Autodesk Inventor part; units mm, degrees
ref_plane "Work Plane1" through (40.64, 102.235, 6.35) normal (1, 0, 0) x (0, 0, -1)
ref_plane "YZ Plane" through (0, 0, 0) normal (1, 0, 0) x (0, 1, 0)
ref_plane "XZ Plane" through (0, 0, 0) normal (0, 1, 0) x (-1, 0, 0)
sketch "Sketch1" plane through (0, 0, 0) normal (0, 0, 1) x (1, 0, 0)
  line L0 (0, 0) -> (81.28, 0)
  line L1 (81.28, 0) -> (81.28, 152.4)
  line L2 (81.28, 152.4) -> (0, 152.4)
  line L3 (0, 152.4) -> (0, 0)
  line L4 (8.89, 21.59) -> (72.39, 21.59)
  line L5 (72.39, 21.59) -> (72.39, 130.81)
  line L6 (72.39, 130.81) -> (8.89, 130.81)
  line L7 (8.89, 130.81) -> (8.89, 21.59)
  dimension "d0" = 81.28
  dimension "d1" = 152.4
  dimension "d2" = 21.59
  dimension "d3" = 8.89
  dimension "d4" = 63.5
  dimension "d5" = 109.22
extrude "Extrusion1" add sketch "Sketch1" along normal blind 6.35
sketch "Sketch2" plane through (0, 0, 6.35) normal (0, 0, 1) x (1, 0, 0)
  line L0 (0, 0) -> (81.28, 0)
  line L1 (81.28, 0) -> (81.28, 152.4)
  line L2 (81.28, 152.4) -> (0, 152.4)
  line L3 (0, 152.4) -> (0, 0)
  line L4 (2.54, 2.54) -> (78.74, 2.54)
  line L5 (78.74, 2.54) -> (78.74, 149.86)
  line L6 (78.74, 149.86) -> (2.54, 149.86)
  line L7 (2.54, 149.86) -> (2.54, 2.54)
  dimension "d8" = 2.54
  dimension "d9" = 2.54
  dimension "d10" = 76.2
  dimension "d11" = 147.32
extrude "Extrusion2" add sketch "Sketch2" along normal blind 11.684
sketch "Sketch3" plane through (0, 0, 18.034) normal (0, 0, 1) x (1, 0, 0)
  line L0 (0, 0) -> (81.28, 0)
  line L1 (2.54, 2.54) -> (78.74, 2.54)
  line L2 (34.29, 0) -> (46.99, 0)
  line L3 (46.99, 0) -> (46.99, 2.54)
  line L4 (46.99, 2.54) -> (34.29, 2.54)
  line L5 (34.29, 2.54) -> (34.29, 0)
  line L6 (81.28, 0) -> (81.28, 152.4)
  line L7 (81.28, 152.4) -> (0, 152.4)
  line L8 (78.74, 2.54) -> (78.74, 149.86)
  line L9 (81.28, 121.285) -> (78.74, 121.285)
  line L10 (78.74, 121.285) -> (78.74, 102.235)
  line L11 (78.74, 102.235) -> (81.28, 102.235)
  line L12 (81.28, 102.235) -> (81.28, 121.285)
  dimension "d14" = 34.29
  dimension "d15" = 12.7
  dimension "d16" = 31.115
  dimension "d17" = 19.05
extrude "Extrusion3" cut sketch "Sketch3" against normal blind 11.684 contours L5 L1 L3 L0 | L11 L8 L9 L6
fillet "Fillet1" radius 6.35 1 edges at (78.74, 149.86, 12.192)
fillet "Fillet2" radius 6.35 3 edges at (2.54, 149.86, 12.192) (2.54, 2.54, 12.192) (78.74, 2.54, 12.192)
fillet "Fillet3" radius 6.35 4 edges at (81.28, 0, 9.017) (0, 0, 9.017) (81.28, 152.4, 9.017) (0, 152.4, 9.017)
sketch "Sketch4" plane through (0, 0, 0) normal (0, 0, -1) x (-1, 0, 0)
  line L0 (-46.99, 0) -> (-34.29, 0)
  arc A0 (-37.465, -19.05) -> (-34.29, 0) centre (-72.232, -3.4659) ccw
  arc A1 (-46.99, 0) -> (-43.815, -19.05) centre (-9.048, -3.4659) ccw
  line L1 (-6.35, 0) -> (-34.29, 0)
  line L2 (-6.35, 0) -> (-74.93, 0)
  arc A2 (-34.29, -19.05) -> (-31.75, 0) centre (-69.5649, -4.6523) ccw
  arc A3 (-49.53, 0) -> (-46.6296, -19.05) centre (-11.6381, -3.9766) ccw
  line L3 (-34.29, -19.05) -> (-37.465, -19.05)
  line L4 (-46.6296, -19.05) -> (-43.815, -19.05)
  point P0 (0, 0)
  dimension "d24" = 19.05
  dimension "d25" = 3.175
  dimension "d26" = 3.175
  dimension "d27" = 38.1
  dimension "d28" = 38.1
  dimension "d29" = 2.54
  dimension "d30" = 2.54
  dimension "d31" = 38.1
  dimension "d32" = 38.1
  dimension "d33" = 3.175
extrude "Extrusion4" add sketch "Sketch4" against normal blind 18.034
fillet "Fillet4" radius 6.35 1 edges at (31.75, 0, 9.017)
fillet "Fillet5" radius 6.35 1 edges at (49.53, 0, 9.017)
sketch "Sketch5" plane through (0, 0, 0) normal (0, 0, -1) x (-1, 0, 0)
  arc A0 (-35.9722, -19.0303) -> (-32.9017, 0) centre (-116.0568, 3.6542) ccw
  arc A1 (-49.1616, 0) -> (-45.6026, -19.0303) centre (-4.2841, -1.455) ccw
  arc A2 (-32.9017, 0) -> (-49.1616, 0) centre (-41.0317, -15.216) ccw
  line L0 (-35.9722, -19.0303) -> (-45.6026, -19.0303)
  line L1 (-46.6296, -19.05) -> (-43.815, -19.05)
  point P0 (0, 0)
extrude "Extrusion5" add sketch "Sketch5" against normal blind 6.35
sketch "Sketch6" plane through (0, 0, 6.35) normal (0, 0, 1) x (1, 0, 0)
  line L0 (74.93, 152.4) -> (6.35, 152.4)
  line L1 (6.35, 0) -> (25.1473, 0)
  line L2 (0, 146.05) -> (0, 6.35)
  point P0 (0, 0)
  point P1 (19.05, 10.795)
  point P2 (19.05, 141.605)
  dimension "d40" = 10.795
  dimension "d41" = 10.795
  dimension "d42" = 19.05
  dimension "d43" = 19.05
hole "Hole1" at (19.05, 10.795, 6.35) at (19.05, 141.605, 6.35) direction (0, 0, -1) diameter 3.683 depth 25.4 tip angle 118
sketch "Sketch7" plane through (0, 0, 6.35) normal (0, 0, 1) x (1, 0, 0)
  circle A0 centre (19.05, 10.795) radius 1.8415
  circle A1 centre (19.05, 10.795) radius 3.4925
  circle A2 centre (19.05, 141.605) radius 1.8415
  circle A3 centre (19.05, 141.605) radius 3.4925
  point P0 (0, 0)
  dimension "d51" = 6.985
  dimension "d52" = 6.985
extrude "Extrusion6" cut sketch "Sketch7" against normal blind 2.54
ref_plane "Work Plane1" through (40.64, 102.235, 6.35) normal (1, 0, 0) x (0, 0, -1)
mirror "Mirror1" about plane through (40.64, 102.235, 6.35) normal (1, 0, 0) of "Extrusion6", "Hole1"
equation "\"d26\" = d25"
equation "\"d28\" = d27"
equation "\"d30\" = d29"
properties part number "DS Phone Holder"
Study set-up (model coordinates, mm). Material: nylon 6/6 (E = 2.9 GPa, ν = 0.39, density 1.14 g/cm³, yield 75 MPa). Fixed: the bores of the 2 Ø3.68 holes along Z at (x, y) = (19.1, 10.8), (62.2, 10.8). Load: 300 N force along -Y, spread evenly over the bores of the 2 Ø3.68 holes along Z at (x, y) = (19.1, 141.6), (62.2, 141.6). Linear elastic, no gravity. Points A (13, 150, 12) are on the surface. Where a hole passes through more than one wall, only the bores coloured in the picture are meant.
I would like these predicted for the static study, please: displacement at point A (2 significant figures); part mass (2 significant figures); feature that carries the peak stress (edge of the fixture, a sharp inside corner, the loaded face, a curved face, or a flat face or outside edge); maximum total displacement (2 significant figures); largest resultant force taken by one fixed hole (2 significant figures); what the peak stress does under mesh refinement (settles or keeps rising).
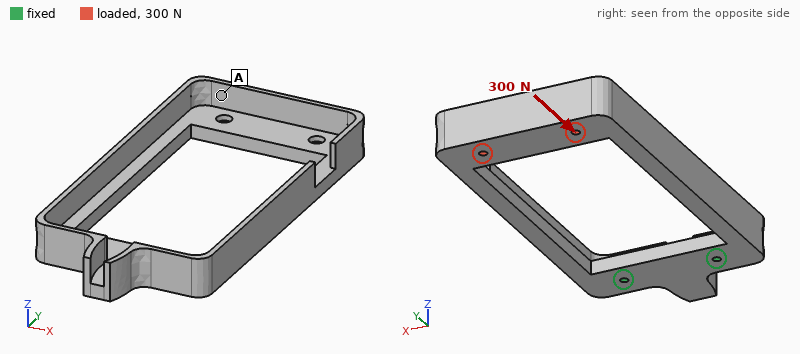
1.1 mm
57 g
edge of the fixture
1.2 mm
150 N
keeps rising
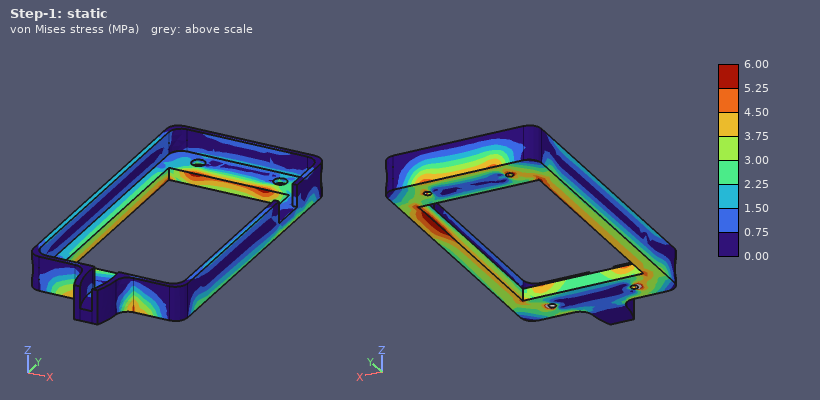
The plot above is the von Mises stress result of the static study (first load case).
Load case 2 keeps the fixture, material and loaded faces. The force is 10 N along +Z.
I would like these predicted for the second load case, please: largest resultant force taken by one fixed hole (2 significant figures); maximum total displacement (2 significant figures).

12 N
2.1 mm
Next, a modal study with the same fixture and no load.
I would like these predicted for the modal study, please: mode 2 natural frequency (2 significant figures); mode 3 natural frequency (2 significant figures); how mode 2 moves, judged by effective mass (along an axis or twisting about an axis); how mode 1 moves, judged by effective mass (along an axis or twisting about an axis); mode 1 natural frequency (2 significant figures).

120 Hz
180 Hz
along X
along Z
78 Hz
